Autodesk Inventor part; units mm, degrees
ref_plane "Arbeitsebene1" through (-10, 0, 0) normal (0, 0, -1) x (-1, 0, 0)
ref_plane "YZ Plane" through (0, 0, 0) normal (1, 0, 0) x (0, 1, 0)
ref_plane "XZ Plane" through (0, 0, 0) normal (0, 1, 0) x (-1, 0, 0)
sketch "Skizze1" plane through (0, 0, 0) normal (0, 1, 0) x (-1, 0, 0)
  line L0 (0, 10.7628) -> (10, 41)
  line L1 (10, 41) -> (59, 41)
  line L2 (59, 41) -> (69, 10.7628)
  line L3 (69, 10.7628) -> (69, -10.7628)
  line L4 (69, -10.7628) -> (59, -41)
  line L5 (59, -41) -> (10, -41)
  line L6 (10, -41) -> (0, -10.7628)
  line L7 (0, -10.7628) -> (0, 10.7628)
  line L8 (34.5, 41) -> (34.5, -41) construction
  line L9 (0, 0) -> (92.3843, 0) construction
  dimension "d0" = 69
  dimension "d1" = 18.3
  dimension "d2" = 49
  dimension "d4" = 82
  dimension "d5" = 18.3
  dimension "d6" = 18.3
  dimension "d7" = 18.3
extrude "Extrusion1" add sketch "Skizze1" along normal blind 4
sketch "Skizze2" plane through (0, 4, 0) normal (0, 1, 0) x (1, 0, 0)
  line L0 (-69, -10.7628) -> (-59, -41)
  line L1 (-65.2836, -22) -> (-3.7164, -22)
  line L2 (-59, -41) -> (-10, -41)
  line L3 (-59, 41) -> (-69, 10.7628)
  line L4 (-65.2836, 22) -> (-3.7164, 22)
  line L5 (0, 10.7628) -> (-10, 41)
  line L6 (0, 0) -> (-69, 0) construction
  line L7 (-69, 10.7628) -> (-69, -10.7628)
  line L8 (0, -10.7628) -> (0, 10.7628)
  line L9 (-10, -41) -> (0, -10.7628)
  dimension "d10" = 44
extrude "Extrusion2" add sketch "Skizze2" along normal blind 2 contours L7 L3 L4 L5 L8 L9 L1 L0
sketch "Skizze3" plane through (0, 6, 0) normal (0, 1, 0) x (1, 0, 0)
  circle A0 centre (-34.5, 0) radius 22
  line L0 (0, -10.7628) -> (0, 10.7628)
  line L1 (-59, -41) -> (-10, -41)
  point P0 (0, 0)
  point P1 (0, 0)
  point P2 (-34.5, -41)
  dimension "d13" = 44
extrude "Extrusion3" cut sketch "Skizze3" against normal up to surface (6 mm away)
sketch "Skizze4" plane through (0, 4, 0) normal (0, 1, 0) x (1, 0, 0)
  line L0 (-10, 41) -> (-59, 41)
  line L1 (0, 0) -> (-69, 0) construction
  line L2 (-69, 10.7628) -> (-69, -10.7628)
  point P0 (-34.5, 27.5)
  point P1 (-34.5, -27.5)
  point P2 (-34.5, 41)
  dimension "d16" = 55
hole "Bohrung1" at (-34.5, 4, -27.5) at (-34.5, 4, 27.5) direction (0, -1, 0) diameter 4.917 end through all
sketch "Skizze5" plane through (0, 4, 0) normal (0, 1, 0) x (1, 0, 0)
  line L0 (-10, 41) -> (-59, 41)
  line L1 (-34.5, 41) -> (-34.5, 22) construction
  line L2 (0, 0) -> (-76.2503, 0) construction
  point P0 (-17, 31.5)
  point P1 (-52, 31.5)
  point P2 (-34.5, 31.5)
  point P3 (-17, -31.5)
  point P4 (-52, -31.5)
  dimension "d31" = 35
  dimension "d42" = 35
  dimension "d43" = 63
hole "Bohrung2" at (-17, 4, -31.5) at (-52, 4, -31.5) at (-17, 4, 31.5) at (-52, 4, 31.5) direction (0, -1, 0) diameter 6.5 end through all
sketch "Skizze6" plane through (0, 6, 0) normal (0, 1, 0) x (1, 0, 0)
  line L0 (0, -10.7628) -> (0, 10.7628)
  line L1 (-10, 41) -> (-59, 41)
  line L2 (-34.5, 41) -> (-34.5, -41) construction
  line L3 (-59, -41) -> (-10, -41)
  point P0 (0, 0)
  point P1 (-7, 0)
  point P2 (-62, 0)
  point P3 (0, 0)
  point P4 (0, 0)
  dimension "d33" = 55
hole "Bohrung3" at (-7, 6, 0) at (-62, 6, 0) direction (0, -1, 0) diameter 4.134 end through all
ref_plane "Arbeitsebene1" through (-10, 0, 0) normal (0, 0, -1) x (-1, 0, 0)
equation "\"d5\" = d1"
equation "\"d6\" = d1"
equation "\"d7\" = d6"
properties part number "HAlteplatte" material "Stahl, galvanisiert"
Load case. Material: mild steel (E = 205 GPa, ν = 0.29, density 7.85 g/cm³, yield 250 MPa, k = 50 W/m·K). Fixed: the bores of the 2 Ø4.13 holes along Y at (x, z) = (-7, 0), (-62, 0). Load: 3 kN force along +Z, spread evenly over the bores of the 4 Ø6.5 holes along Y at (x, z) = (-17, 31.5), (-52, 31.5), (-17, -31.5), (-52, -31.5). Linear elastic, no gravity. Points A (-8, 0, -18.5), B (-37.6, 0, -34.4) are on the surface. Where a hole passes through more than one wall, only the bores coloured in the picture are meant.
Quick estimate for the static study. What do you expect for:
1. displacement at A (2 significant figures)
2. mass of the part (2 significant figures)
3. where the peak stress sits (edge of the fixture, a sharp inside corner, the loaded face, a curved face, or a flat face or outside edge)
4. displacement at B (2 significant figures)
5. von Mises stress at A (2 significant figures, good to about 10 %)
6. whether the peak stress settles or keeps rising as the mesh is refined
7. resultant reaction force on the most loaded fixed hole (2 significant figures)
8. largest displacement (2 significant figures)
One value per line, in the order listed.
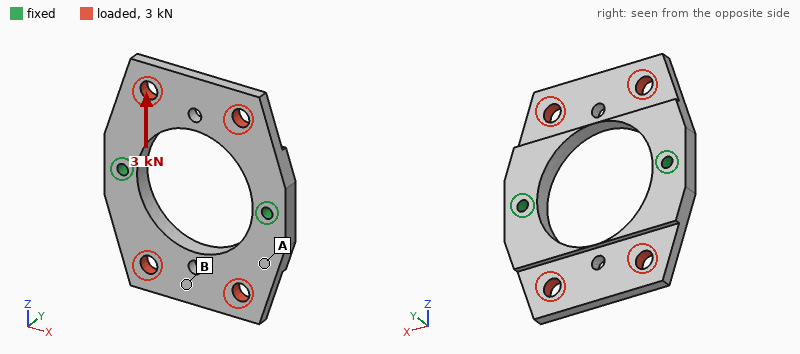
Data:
3.1 µm
130 g
edge of the fixture
9.4 µm
15 MPa
keeps rising
1.5 kN
11 µm
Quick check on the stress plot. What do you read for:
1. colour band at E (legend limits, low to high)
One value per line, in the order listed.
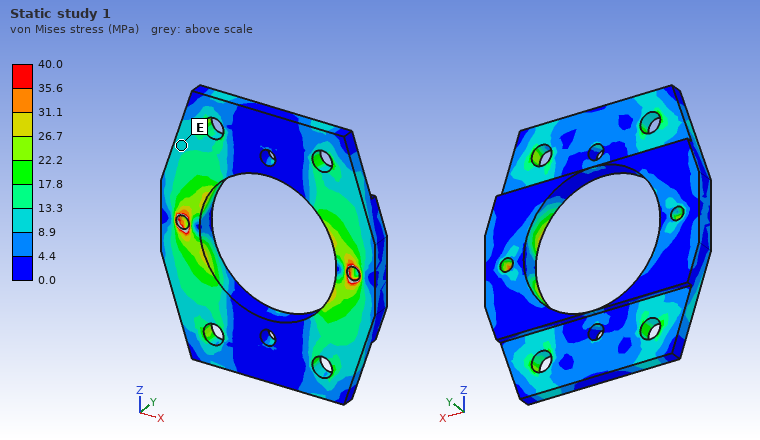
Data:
8.9 to 13.3 MPa
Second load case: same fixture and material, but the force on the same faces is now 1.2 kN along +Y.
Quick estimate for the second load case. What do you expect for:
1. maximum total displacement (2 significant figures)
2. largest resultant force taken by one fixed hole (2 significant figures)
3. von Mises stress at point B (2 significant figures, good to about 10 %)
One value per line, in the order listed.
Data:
0.11 mm
600 N
16 MPa
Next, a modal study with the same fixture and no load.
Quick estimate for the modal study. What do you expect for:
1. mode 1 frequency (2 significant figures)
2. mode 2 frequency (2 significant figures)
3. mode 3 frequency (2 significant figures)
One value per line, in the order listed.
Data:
2300 Hz
2400 Hz
5000 Hz
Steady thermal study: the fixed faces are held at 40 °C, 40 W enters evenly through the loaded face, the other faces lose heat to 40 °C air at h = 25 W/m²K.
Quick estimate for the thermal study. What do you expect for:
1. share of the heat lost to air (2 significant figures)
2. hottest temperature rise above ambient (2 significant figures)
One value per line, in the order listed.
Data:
24 %
71 K
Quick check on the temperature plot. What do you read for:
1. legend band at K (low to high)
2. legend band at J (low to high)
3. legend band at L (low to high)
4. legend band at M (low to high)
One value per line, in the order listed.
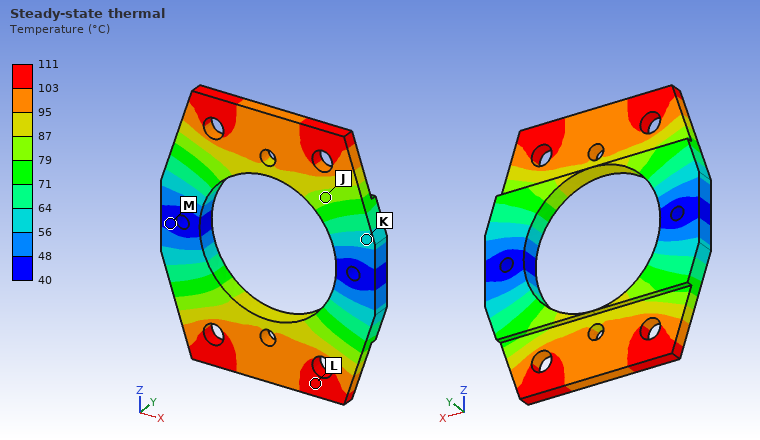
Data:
56 to 64 °C
79 to 87 °C
103 to 111 °C
40 to 48 °C
